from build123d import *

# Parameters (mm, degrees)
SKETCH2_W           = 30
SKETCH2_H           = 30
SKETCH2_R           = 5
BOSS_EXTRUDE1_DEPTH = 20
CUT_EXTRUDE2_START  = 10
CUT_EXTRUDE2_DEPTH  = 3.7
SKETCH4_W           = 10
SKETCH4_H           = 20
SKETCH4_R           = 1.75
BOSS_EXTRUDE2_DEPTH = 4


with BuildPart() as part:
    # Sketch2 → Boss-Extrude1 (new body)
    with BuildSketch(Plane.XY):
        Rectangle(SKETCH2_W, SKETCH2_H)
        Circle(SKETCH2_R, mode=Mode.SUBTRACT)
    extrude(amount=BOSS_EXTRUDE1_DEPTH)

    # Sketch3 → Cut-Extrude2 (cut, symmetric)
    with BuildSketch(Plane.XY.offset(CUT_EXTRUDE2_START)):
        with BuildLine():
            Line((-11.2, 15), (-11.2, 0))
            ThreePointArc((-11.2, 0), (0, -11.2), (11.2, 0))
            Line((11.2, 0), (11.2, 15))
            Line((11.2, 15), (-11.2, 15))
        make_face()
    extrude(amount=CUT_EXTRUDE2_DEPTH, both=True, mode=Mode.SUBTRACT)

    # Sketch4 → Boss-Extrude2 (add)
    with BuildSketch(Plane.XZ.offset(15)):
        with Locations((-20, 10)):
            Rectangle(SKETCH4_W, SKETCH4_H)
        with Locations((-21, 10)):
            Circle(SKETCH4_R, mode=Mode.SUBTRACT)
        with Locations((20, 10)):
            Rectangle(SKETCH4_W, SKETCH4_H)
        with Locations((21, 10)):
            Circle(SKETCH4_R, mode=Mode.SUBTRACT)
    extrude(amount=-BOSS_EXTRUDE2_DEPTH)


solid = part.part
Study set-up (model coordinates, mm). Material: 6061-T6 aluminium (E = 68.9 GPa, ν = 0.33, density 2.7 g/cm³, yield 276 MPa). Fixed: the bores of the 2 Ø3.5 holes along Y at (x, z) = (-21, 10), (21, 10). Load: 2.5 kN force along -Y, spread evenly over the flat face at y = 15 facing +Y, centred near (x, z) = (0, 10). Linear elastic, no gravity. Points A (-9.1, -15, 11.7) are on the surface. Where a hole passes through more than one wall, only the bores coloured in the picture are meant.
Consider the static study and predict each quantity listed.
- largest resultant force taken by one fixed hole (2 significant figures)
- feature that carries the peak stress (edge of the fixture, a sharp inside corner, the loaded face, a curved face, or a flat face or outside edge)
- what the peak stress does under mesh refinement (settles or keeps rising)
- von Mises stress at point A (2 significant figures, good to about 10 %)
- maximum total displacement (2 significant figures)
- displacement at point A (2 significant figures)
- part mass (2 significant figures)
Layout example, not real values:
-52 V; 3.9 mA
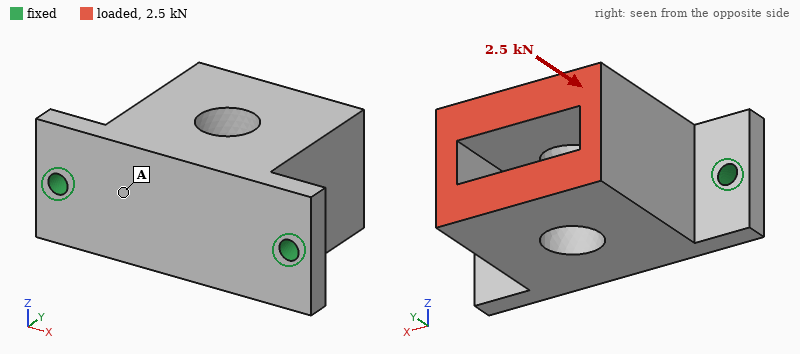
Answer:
1.3 kN; edge of the fixture; keeps rising; 16 MPa; 20 µm; 18 µm; 39 g
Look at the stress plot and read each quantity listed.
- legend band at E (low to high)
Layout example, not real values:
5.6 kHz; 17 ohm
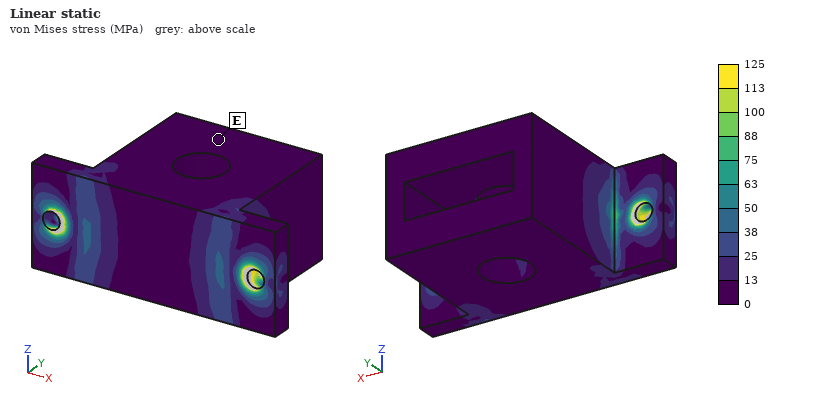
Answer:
0 to 13 MPa
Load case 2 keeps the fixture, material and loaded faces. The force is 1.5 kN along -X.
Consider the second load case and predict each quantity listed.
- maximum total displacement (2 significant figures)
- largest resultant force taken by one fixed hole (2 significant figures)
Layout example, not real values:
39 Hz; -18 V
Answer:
40 µm; 1.4 kN
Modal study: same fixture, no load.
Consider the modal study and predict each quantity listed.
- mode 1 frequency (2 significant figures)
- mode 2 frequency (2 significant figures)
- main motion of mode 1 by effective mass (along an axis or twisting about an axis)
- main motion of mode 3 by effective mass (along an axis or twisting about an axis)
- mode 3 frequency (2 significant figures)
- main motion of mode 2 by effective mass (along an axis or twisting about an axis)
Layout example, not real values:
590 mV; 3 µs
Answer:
2800 Hz; 9100 Hz; along Z; along Y; 9600 Hz; along X
